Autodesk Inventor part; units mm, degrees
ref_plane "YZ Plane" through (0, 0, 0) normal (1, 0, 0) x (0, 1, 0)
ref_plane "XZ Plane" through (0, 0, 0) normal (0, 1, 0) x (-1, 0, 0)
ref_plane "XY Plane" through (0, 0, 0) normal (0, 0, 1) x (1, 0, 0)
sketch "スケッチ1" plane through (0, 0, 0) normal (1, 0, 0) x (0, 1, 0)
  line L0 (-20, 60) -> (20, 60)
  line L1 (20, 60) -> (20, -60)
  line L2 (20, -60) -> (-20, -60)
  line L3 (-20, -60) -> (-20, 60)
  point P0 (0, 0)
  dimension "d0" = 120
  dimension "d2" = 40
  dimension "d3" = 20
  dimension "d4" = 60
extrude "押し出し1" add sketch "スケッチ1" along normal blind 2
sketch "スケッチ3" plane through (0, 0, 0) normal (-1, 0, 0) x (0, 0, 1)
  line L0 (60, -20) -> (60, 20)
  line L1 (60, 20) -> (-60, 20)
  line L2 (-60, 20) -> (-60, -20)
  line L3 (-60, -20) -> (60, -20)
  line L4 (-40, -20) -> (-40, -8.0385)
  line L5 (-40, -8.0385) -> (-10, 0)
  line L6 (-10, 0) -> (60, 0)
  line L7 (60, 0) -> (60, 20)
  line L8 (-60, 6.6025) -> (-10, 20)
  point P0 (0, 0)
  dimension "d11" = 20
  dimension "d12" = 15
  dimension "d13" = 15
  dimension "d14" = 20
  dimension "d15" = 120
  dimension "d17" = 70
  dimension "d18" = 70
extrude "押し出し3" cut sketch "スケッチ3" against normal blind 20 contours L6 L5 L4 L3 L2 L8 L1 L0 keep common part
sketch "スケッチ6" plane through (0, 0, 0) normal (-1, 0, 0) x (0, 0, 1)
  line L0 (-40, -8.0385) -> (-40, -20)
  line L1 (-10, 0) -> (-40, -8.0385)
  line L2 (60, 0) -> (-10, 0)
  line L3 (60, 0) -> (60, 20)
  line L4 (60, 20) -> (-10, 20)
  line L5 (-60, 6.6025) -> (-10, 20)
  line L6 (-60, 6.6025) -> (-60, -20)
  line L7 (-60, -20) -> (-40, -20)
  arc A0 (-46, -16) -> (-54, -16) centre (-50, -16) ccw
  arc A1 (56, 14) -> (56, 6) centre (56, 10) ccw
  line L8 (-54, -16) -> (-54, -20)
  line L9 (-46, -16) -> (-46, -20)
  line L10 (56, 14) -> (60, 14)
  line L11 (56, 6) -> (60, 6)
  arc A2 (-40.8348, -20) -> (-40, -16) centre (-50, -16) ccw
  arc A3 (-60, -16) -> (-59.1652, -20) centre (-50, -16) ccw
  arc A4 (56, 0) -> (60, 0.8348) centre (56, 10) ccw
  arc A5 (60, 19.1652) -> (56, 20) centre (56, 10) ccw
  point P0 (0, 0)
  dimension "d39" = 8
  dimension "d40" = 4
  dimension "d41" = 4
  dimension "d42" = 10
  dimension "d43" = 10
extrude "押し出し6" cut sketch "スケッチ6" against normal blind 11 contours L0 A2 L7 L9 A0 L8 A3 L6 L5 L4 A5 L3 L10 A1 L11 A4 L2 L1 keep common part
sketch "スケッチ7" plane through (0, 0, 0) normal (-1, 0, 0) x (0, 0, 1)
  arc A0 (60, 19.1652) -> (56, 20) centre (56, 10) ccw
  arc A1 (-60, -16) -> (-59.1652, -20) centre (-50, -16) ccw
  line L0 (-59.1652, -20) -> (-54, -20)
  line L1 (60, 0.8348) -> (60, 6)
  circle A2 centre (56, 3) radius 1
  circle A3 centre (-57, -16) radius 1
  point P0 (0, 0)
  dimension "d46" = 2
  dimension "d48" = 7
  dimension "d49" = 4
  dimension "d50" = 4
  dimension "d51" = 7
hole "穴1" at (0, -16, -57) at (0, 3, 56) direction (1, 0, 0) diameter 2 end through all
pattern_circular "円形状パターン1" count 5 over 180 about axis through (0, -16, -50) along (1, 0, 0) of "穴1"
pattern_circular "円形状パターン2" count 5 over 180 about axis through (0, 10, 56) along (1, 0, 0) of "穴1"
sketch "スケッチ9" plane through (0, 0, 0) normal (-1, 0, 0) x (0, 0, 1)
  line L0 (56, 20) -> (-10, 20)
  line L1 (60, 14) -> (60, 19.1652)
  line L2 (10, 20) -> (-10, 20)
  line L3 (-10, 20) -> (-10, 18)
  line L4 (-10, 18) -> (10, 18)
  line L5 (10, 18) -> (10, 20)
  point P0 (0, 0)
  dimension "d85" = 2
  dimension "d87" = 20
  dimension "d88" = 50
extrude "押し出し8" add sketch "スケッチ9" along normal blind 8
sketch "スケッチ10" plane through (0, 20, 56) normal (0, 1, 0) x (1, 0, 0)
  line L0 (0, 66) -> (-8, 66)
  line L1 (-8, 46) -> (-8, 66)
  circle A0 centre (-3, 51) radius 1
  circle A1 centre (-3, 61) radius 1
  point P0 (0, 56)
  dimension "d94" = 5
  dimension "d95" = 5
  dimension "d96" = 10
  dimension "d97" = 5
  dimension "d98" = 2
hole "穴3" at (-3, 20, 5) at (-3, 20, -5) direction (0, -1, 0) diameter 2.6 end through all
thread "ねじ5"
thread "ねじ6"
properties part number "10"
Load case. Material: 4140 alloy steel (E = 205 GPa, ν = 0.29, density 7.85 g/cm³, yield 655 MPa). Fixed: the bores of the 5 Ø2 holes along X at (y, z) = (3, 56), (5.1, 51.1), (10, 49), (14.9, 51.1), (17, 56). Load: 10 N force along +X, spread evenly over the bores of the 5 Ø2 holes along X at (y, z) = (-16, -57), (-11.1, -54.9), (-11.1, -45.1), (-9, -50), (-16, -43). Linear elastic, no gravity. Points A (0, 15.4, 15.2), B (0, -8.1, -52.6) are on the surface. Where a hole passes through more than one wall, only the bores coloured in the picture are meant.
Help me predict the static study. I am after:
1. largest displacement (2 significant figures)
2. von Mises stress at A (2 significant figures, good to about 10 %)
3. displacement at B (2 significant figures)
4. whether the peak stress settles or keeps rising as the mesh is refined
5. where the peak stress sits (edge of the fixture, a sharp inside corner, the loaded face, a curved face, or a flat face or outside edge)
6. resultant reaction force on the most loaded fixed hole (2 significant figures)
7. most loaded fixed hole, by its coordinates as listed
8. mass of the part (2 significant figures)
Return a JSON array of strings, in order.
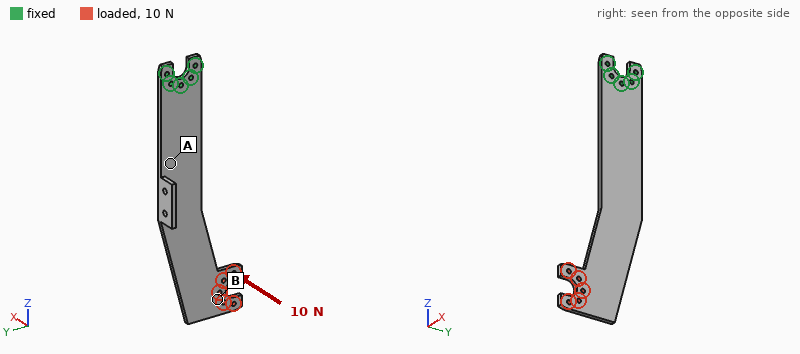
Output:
["1.4 mm", "52 MPa", "1.2 mm", "keeps rising", "edge of the fixture", "94 N", "(10, 49)", "41 g"]
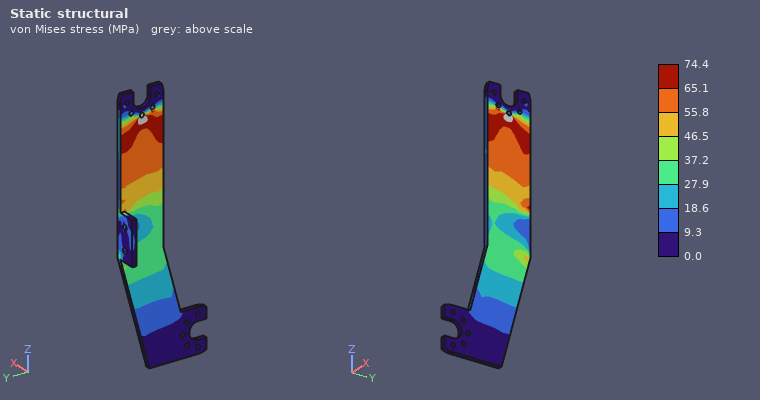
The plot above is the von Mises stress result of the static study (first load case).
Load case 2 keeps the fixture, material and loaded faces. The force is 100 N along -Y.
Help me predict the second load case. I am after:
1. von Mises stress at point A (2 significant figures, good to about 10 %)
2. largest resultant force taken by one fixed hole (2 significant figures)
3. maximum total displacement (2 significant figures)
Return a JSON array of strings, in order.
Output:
["27 MPa", "520 N", "0.16 mm"]
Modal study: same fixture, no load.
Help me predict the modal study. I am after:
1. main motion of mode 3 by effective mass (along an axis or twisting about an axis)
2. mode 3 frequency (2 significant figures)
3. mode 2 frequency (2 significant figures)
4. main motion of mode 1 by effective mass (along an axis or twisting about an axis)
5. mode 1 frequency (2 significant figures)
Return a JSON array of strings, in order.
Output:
["along Y", "1200 Hz", "720 Hz", "along X", "130 Hz"]
